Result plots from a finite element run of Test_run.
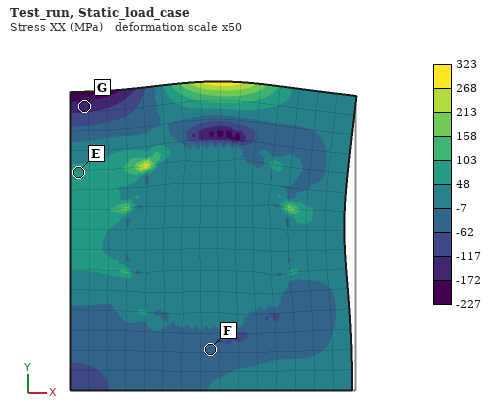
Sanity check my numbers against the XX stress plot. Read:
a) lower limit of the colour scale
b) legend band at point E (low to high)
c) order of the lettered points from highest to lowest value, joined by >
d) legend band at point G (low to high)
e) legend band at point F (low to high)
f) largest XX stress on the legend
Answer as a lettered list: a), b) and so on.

a) -227 MPa
b) 48 to 103 MPa
c) E > F > G
d) -172 to -117 MPa
e) -62 to -7 MPa
f) 323 MPa
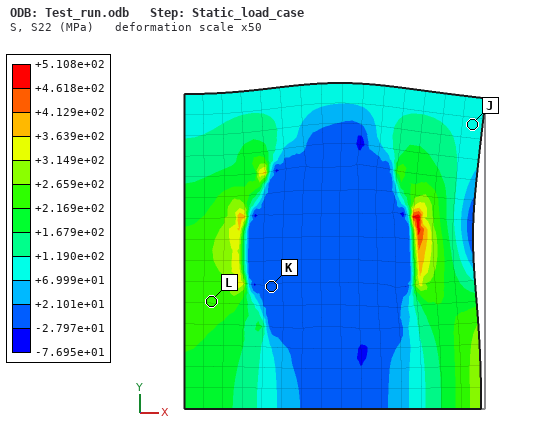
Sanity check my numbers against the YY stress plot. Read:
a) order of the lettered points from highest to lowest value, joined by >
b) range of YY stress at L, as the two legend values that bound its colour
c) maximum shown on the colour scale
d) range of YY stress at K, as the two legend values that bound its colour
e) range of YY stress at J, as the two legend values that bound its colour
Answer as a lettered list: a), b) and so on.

a) L > J > K
b) +2.169e+02 to +2.659e+02 MPa
c) +5.108e+02 MPa
d) -2.797e+01 to +2.101e+01 MPa
e) +6.999e+01 to +1.190e+02 MPa
